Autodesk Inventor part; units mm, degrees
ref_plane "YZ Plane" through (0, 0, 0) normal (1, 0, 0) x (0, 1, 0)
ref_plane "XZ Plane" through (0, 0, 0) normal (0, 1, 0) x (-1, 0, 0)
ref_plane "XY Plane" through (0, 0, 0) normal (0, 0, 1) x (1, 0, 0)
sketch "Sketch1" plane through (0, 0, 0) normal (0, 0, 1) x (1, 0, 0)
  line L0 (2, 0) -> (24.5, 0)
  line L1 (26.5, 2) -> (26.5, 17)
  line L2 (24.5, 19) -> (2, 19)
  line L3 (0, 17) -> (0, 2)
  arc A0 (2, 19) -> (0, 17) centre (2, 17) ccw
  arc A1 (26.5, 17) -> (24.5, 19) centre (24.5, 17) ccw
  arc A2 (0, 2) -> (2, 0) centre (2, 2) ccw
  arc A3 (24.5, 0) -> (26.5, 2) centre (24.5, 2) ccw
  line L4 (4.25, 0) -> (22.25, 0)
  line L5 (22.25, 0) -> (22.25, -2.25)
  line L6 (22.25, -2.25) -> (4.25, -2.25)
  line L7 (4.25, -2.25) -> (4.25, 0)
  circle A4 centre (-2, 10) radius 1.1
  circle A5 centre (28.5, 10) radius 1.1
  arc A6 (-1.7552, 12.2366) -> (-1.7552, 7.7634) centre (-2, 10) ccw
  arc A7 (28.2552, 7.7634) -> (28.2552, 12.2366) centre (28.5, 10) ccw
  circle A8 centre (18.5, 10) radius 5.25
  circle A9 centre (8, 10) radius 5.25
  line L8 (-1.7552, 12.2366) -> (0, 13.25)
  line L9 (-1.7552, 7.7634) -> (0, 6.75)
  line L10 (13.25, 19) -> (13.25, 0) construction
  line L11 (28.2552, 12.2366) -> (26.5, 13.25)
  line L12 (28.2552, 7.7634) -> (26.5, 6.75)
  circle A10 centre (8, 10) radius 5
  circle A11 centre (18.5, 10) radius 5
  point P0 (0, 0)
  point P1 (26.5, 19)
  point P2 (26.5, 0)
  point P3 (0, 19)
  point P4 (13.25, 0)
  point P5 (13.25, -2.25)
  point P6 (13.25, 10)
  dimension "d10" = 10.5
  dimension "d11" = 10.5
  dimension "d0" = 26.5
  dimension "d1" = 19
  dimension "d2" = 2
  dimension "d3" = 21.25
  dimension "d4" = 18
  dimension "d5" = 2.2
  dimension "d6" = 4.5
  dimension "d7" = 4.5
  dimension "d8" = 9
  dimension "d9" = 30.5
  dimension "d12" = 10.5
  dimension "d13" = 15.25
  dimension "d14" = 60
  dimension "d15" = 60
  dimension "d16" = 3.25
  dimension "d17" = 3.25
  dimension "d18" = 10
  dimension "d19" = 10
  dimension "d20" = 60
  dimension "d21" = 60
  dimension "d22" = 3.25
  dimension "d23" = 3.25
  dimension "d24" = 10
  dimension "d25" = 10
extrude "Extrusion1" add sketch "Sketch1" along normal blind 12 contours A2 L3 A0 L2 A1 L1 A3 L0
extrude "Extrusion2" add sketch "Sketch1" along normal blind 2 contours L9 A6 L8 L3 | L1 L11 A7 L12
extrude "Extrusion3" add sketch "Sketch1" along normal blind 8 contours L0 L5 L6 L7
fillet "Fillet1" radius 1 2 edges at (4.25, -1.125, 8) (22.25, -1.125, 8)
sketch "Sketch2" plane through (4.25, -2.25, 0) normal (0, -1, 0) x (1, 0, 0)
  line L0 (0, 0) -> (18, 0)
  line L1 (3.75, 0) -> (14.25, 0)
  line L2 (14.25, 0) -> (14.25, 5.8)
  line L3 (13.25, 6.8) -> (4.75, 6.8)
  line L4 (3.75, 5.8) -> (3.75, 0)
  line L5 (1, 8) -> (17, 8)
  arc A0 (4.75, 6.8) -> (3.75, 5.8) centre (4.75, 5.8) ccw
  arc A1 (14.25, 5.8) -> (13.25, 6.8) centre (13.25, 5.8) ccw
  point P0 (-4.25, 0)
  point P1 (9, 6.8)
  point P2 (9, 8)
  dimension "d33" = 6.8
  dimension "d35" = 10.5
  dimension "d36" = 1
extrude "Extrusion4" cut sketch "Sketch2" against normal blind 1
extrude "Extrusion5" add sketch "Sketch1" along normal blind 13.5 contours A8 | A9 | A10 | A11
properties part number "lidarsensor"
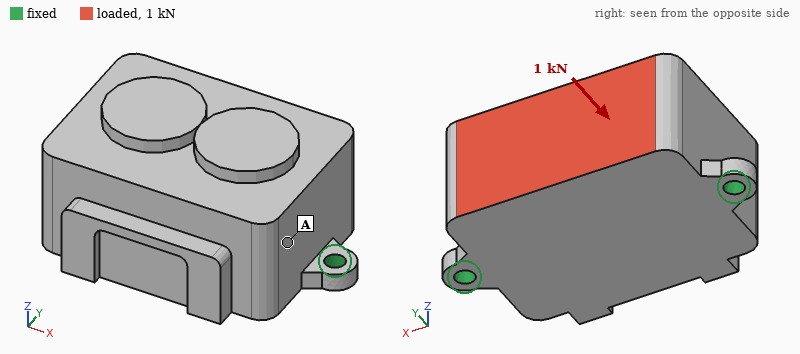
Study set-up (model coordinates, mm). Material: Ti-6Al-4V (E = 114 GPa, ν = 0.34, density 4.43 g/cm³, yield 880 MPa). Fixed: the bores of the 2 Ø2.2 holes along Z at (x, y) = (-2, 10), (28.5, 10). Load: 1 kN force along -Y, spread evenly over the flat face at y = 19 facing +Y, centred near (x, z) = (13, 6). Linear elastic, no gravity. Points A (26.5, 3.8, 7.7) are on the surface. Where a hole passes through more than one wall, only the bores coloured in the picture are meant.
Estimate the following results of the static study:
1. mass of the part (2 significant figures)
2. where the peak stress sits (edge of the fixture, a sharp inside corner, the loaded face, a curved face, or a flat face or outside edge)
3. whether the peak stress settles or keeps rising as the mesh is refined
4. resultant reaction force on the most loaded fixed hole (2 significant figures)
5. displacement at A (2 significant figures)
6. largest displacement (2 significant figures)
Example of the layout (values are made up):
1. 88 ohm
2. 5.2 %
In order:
1. 29 g
2. edge of the fixture
3. keeps rising
4. 500 N
5. 0.072 mm
6. 0.12 mm
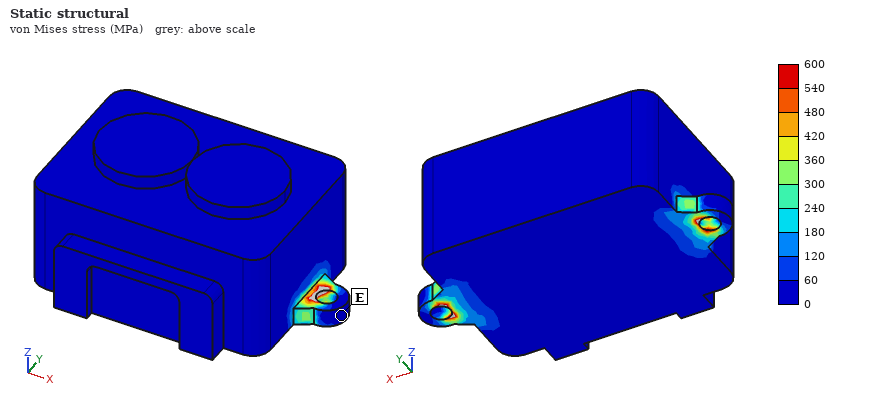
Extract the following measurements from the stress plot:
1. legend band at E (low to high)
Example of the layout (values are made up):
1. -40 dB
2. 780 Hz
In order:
1. 0 to 60 MPa
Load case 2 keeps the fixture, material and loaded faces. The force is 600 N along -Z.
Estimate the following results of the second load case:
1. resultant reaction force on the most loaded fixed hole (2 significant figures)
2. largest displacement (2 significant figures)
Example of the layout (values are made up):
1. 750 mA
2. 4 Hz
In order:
1. 350 N
2. 0.12 mm
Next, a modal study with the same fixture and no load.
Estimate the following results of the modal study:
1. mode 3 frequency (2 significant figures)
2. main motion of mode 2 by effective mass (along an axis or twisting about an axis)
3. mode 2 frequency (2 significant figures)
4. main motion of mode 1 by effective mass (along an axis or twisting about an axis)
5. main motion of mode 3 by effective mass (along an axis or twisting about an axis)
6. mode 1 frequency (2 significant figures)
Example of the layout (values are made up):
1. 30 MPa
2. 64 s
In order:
1. 18 kHz
2. along Z
3. 13 kHz
4. along Y
5. along X
6. 2800 Hz
